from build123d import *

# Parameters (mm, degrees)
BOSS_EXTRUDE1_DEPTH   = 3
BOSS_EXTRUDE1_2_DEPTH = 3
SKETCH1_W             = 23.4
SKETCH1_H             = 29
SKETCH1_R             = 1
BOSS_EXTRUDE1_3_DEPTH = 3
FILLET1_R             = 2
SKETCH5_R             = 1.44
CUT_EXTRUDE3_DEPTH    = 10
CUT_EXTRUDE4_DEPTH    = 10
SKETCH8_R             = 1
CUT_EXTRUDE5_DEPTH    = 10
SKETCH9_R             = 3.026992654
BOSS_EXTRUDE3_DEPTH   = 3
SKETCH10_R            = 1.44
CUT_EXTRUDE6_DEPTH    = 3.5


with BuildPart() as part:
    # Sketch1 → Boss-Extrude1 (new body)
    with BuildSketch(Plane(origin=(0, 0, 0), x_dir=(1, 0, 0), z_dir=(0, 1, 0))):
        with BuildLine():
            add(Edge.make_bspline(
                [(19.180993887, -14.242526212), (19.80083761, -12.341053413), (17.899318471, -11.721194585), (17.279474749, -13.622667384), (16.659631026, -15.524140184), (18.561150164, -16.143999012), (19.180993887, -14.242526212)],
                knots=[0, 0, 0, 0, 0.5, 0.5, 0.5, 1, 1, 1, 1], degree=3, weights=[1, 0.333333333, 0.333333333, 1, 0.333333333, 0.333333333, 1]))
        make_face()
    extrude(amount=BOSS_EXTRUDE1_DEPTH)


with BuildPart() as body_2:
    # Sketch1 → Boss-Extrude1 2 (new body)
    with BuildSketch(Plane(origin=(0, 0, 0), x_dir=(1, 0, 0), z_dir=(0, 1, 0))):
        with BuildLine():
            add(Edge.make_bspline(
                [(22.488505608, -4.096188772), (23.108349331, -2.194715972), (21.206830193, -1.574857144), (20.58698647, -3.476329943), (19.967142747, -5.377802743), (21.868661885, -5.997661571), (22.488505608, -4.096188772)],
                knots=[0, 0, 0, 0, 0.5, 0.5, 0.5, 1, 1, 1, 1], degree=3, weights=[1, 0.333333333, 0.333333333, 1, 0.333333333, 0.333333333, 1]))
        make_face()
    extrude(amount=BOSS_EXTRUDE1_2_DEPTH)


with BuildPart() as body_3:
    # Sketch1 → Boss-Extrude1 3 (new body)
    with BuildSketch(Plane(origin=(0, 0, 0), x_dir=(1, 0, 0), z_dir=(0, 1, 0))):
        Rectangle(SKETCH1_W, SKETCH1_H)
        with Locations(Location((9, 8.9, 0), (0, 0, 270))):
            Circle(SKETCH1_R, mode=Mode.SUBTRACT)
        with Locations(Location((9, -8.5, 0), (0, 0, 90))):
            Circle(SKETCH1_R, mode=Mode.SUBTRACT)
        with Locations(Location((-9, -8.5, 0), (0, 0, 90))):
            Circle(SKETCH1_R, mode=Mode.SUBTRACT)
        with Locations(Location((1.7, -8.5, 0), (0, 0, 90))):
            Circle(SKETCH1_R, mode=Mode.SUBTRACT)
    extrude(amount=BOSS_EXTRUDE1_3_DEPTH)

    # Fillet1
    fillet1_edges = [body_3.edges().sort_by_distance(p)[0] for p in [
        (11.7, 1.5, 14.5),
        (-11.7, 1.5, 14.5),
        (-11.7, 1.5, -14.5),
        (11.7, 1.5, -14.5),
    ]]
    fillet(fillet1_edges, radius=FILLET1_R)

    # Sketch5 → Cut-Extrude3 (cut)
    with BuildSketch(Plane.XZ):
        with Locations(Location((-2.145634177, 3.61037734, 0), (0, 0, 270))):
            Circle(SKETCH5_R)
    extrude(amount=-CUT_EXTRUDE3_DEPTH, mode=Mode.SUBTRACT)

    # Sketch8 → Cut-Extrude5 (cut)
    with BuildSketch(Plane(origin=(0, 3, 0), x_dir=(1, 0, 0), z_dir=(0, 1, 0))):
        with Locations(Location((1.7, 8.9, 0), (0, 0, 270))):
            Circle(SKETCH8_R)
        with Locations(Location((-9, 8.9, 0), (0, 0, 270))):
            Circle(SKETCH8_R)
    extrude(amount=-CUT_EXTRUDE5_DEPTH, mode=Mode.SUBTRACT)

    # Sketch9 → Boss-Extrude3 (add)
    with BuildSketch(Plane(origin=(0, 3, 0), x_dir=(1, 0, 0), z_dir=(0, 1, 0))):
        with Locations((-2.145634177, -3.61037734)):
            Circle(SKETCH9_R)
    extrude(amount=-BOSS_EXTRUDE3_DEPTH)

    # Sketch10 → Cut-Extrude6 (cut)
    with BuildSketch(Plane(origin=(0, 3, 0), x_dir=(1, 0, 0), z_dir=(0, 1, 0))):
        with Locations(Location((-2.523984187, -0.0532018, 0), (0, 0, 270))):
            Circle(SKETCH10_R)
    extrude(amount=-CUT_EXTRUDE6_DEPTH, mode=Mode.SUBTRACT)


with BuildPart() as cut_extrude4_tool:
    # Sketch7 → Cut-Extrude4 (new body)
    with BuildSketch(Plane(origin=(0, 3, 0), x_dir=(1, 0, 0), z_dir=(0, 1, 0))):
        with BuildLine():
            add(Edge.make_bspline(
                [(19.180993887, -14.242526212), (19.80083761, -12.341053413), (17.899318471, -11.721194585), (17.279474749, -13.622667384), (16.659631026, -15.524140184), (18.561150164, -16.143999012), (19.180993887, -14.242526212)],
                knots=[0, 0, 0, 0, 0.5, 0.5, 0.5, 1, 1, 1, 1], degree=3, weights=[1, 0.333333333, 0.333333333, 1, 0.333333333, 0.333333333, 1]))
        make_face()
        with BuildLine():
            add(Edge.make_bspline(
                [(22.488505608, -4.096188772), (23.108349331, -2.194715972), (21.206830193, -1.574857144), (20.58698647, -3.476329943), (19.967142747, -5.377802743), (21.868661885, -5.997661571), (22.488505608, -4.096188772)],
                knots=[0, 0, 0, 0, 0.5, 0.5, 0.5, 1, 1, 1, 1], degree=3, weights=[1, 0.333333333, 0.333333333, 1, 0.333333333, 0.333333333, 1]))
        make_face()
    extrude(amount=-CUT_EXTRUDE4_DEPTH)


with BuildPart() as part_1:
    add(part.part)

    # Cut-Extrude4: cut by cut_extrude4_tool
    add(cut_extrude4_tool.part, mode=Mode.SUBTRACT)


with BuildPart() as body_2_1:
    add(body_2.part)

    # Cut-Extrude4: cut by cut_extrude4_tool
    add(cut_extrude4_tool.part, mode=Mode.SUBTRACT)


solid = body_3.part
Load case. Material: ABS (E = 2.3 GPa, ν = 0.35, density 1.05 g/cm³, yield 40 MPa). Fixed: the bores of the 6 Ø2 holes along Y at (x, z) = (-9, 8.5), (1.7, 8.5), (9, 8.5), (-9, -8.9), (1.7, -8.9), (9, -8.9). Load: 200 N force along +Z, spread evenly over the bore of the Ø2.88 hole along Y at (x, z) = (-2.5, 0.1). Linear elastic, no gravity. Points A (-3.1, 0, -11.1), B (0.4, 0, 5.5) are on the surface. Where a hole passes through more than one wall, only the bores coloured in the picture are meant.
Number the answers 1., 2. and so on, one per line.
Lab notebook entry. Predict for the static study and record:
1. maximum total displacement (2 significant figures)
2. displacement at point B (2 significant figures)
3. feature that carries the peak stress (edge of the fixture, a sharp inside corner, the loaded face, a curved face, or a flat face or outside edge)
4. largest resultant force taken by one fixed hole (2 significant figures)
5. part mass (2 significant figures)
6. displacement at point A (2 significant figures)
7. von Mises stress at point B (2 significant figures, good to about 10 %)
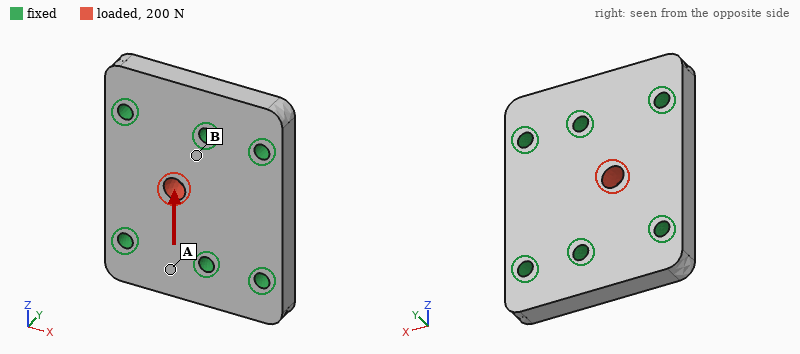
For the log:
1. 17 µm
2. 4.4 µm
3. the loaded face
4. 53 N
5. 2.0 g
6. 3.8 µm
7. 3.9 MPa
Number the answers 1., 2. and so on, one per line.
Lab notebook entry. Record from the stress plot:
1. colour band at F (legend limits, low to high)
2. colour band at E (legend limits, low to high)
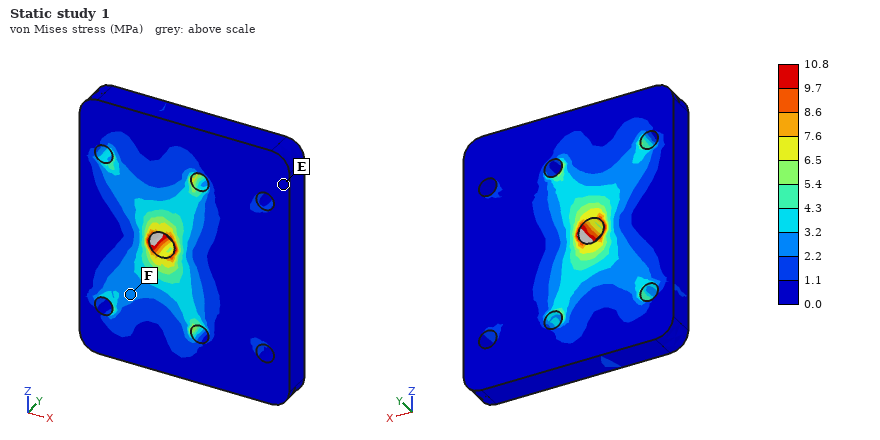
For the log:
1. 2.2 to 3.2 MPa
2. 0.0 to 1.1 MPa
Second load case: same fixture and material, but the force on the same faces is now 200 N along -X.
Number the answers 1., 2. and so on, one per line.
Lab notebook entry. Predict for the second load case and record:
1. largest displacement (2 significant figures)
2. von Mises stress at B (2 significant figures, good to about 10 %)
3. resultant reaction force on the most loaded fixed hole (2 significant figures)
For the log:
1. 23 µm
2. 3.4 MPa
3. 45 N
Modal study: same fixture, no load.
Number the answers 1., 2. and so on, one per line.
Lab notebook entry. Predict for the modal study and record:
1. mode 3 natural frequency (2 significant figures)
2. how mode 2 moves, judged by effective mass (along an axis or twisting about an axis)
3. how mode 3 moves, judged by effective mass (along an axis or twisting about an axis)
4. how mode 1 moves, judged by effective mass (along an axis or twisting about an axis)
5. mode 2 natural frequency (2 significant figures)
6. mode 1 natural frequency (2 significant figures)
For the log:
1. 17 kHz
2. twisting about Z
3. along Y
4. along Y
5. 15 kHz
6. 13 kHz
